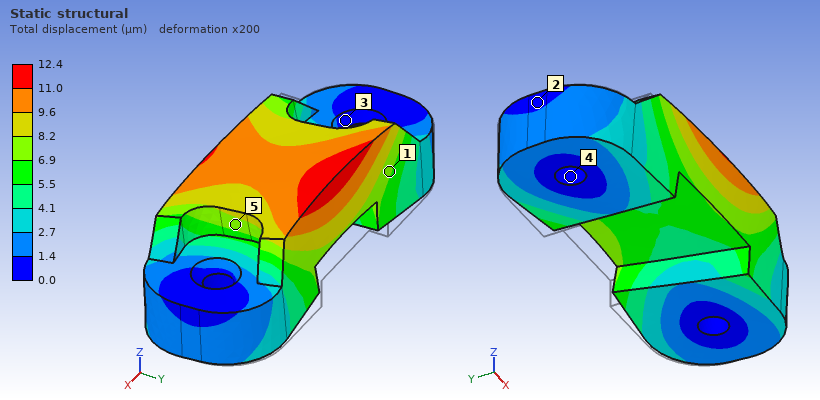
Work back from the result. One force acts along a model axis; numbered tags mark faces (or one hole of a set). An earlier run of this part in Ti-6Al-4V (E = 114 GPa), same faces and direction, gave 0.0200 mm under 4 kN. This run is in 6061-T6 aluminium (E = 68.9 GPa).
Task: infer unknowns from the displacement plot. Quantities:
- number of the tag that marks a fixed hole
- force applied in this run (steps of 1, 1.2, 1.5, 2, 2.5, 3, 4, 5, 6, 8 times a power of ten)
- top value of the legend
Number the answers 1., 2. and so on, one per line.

1. 4
2. 1.5 kN
3. 12.4 µm
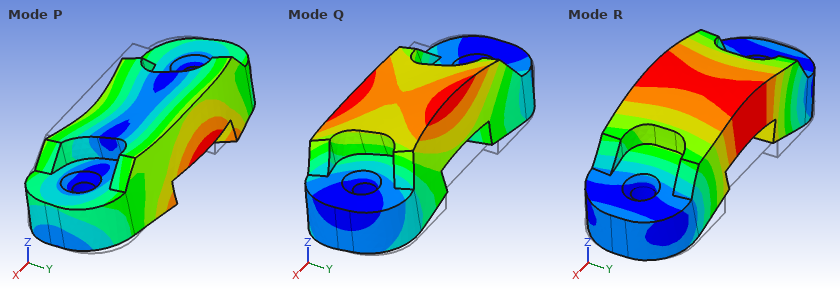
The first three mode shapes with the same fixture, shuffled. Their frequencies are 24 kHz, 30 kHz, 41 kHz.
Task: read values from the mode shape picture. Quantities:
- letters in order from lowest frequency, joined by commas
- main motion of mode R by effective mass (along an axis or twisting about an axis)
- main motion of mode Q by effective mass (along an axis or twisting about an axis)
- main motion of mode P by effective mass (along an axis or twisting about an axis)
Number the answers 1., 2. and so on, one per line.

1. Q, R, P
2. along Z
3. along Y
4. along Y
